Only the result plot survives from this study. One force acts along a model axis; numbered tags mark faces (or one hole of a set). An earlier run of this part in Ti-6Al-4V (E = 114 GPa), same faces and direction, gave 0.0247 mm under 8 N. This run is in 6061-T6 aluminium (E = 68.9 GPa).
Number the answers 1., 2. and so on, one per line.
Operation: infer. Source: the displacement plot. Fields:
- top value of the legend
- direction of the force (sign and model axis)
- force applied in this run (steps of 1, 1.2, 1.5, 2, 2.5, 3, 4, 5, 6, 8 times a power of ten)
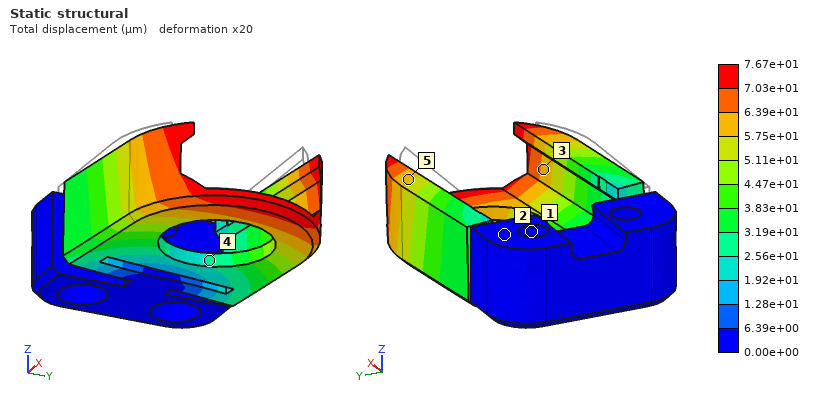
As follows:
1. 7.67e+01 µm
2. +Y
3. 15 N
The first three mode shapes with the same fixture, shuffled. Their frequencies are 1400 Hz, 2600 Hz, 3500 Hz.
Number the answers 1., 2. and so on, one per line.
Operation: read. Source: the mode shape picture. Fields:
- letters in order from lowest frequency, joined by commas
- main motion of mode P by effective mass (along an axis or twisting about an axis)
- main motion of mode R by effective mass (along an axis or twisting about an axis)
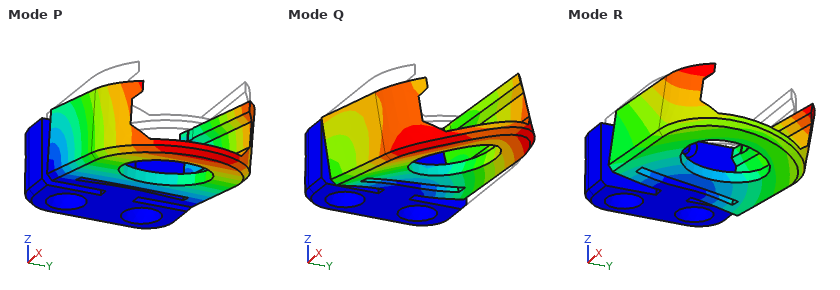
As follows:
1. P, R, Q
2. along Z
3. along Y
